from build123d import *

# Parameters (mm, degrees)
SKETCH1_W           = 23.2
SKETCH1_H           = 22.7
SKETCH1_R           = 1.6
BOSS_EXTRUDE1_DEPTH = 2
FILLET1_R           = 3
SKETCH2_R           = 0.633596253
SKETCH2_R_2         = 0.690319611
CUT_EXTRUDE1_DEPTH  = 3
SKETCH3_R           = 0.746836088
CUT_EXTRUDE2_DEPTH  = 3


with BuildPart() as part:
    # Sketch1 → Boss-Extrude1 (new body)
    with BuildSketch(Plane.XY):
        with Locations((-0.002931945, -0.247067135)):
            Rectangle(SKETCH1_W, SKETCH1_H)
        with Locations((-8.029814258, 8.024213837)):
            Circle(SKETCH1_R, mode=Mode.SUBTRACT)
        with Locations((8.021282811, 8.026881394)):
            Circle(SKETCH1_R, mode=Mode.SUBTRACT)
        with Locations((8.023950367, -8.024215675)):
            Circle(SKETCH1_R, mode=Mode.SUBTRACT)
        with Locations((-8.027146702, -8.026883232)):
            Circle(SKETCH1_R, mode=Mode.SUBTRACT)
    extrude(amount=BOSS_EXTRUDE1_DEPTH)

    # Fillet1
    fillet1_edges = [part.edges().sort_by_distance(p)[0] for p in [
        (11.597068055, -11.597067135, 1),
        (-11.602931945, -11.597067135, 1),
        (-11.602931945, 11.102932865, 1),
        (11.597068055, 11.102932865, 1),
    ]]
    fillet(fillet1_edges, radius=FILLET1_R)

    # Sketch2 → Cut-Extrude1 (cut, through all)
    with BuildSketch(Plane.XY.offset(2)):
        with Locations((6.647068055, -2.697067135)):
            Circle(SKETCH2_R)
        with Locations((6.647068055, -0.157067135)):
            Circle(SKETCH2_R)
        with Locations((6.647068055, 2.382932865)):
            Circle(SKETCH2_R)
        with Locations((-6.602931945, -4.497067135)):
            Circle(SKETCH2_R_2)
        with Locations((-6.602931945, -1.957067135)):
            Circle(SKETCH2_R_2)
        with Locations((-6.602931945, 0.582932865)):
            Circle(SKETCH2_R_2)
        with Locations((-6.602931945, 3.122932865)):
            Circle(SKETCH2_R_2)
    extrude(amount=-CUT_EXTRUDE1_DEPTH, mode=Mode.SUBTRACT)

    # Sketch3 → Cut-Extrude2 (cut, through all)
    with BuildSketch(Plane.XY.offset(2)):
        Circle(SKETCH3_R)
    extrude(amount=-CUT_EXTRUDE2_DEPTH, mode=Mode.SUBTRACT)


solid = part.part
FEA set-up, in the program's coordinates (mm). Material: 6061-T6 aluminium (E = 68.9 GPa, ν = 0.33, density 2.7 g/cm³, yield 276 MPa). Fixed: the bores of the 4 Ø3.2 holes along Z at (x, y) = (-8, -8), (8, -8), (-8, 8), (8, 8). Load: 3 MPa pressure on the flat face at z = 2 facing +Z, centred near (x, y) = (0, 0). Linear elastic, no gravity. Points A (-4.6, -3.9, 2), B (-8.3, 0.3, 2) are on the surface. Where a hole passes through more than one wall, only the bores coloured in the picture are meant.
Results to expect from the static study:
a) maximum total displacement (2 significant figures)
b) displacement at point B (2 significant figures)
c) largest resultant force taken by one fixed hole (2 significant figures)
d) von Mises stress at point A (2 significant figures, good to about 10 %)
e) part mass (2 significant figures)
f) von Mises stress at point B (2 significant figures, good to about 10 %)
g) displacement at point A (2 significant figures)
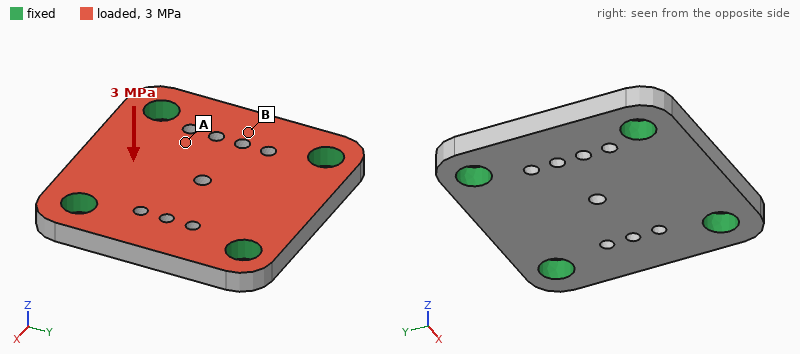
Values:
19 µm
9.8 µm
370 N
17 MPa
2.6 g
43 MPa
11 µm
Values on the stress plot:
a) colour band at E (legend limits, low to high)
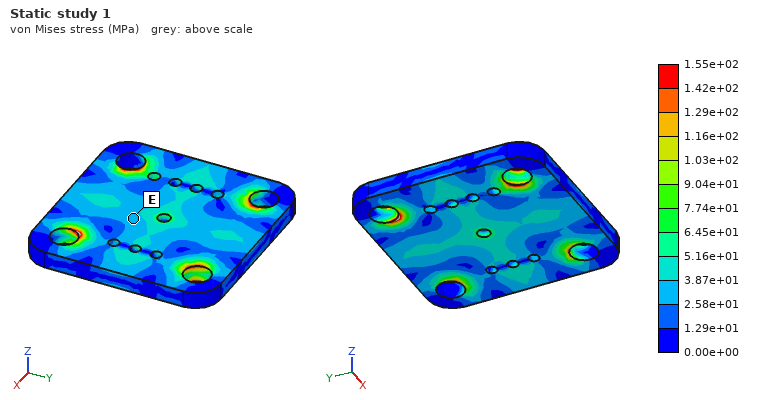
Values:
2.58e+01 to 3.87e+01 MPa
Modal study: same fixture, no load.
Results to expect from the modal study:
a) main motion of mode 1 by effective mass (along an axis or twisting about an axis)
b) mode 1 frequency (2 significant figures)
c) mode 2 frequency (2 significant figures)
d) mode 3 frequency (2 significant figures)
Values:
along Z
33 kHz
49 kHz
49 kHz
